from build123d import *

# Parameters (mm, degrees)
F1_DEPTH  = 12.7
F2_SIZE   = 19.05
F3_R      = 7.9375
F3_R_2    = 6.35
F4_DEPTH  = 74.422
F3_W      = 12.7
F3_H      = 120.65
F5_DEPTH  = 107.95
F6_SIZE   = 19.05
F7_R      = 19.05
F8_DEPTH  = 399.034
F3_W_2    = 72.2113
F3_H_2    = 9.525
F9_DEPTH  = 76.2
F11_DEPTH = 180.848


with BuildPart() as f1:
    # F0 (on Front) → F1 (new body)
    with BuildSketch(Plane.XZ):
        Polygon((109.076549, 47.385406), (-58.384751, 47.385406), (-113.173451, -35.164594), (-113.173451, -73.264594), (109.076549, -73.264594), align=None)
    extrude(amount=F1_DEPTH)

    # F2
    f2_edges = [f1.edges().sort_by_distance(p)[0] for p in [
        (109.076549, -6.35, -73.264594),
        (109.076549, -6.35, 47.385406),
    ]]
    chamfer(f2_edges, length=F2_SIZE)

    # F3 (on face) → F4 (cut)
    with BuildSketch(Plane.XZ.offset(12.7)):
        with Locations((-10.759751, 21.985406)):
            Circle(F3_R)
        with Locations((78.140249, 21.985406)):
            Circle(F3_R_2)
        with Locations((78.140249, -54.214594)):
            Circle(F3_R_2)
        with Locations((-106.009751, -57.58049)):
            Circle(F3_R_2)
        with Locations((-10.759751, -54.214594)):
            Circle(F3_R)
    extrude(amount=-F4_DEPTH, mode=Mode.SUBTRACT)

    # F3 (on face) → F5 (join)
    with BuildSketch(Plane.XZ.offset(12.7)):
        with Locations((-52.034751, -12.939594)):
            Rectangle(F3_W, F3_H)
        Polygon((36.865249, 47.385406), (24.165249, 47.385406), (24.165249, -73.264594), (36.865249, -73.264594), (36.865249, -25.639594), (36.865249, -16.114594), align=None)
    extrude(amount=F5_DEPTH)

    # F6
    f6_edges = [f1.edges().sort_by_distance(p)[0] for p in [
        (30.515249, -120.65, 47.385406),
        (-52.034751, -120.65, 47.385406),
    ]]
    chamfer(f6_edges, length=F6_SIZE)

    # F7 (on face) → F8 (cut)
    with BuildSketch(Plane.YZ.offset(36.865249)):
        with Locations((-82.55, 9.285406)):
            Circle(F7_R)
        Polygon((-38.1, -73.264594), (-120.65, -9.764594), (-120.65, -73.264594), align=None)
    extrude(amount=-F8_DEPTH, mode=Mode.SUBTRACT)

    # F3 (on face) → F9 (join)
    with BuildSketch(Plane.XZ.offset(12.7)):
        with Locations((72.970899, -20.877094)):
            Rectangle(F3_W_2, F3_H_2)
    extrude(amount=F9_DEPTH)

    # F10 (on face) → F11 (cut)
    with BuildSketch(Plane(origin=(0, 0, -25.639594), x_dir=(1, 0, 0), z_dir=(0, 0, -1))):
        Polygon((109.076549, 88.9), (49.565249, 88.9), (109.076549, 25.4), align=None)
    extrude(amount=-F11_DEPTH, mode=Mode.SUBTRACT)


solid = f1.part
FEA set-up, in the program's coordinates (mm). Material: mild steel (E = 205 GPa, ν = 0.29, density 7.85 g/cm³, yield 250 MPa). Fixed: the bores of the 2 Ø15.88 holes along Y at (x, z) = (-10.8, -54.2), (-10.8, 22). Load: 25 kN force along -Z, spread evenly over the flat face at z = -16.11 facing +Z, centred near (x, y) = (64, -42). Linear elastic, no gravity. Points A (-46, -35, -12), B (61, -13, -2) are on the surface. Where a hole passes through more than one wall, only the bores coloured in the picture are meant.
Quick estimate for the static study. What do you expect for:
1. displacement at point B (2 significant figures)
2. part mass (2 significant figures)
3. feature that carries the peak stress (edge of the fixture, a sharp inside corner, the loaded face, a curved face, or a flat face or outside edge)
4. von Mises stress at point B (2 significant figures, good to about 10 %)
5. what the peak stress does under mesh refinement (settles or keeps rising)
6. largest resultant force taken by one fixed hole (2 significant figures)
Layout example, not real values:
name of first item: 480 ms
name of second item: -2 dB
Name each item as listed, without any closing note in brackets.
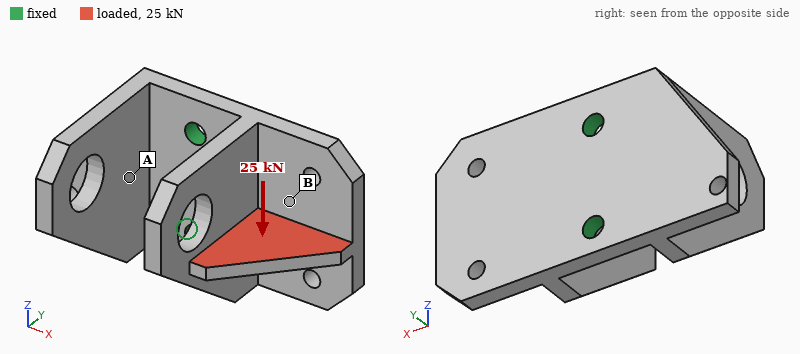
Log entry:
displacement at point B: 0.040 mm
part mass: 4.4 kg
feature that carries the peak stress: edge of the fixture
von Mises stress at point B: 58 MPa
what the peak stress does under mesh refinement: keeps rising
largest resultant force taken by one fixed hole: 28 kN
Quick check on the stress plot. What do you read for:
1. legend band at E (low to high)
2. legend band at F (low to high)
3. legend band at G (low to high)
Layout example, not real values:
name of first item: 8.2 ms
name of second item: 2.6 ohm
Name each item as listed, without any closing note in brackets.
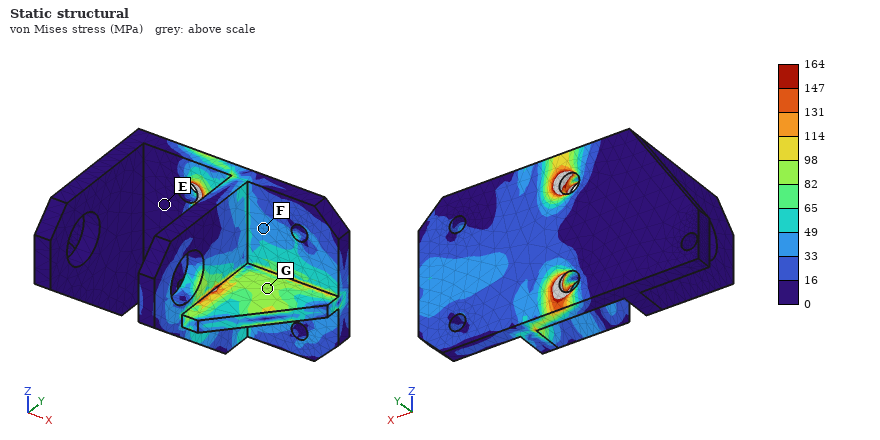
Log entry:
legend band at E: 0 to 16 MPa
legend band at F: 33 to 49 MPa
legend band at G: 82 to 98 MPa
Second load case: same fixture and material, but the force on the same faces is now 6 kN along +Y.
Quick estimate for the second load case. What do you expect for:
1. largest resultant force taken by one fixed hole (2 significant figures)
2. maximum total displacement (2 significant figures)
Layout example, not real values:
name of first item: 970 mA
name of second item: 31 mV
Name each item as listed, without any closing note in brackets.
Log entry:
largest resultant force taken by one fixed hole: 3.1 kN
maximum total displacement: 0.36 mm
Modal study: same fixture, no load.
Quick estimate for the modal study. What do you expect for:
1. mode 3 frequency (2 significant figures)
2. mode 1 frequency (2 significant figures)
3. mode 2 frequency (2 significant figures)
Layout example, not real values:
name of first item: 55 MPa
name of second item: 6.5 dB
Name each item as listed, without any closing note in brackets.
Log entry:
mode 3 frequency: 1600 Hz
mode 1 frequency: 560 Hz
mode 2 frequency: 690 Hz
